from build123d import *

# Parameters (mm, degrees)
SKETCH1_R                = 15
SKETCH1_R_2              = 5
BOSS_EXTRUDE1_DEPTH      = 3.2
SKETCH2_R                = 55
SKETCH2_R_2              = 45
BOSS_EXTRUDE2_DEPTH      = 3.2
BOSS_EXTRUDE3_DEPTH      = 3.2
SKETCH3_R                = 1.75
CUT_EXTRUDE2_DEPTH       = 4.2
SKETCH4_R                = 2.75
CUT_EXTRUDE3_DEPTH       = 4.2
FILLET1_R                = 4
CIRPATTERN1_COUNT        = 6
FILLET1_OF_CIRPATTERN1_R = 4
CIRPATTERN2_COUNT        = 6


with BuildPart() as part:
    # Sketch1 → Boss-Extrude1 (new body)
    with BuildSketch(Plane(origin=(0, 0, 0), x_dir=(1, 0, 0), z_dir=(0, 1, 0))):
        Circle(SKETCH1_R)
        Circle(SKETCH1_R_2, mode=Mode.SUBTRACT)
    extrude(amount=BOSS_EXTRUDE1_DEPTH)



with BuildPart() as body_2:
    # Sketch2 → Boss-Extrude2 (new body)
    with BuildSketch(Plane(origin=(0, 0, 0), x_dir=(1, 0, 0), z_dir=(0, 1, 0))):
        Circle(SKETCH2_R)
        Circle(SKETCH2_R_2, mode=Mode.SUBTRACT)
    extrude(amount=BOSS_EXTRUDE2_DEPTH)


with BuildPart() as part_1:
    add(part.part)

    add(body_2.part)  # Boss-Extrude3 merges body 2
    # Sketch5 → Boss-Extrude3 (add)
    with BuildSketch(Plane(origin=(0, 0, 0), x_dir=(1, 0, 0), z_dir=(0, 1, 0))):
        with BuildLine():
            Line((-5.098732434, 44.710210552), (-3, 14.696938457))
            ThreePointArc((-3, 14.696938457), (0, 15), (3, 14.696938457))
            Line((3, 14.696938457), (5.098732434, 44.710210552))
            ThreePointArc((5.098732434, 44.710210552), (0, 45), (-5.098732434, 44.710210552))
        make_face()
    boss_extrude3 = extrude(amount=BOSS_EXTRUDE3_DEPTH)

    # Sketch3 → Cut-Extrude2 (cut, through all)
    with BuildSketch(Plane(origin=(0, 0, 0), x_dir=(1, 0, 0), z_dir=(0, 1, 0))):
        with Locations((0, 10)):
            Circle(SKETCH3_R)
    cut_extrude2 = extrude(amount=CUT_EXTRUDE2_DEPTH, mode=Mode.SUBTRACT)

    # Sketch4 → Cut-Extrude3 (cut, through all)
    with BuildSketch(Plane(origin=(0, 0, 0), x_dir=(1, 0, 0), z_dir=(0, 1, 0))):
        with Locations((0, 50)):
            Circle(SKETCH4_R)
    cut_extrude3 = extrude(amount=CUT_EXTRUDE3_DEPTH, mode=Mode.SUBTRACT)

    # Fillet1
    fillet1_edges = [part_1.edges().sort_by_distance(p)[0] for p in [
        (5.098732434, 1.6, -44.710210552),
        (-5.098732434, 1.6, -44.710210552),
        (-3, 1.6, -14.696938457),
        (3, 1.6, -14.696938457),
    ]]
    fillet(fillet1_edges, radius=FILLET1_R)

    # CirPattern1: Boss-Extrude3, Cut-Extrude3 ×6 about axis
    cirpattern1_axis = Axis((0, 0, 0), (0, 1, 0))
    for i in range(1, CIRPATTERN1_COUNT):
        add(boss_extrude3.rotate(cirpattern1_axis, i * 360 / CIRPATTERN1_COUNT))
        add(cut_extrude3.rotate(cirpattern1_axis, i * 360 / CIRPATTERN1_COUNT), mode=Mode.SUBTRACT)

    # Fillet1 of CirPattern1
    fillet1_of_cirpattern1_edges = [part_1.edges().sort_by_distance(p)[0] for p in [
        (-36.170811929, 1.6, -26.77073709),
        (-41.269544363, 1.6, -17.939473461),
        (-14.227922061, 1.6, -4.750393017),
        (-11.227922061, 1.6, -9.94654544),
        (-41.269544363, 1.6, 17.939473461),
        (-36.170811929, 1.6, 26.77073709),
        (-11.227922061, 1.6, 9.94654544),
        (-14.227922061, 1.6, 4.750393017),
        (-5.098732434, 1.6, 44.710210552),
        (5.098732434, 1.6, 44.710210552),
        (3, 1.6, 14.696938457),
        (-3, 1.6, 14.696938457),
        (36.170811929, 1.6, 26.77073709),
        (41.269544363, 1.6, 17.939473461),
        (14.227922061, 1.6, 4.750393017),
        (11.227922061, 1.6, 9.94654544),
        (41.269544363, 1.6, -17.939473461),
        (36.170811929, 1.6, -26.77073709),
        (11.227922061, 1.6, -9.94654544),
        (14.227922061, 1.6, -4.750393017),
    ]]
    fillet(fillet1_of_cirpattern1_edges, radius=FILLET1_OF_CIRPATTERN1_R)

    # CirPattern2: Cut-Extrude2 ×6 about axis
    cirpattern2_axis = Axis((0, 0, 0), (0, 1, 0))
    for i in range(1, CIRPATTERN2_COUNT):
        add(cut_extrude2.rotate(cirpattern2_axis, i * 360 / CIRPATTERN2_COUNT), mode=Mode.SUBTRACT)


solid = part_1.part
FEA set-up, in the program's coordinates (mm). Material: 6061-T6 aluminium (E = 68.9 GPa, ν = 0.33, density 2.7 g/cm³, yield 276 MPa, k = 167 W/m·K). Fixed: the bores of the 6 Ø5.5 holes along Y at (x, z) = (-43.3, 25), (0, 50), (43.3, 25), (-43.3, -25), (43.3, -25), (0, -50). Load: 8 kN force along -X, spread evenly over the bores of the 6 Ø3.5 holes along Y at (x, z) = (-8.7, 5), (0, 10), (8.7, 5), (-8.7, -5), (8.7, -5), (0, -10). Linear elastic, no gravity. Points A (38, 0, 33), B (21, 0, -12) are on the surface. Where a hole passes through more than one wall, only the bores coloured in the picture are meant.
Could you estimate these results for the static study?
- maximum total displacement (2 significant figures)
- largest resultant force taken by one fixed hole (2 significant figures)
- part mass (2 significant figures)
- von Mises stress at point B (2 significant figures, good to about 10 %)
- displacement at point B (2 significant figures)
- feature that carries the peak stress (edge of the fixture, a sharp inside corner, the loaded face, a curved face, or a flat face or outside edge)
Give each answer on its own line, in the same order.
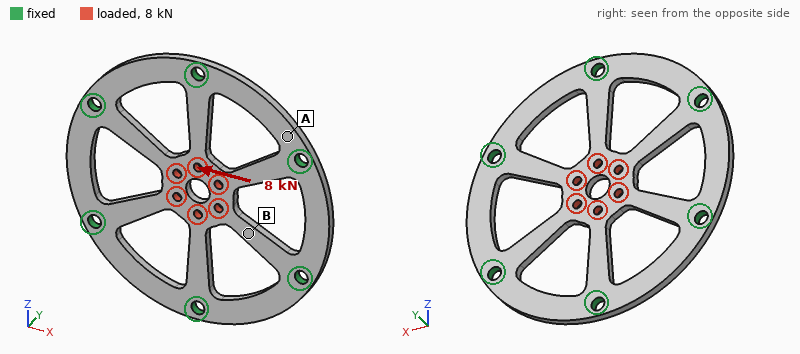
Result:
56 µm
2.1 kN
44 g
93 MPa
31 µm
a sharp inside corner
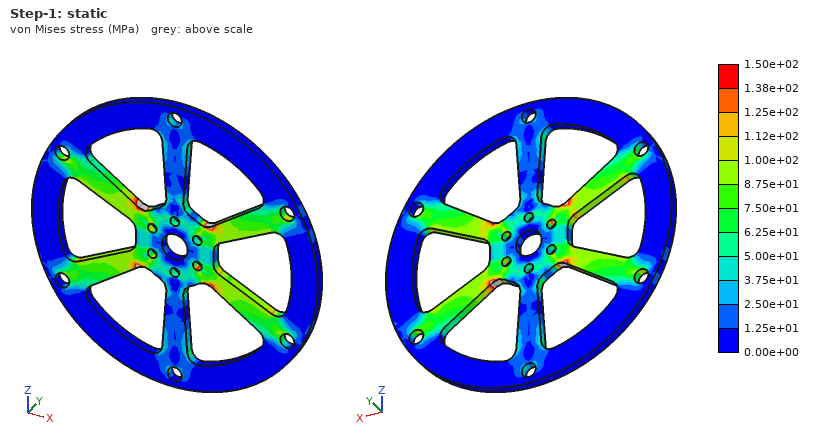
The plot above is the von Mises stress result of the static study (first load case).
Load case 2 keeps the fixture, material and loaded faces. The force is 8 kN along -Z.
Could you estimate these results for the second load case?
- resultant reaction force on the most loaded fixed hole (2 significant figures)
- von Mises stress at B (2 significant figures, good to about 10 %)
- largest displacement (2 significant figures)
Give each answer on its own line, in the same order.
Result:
2.4 kN
55 MPa
55 µm
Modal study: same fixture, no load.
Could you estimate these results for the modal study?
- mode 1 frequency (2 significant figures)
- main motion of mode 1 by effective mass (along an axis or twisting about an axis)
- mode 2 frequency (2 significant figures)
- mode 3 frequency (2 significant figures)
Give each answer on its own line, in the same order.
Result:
2400 Hz
along Y
5500 Hz
5500 Hz
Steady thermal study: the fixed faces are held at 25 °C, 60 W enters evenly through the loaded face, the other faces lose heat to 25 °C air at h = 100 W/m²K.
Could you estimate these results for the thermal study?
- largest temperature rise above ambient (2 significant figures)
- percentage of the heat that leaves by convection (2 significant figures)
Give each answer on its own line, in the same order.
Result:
67 K
33 %
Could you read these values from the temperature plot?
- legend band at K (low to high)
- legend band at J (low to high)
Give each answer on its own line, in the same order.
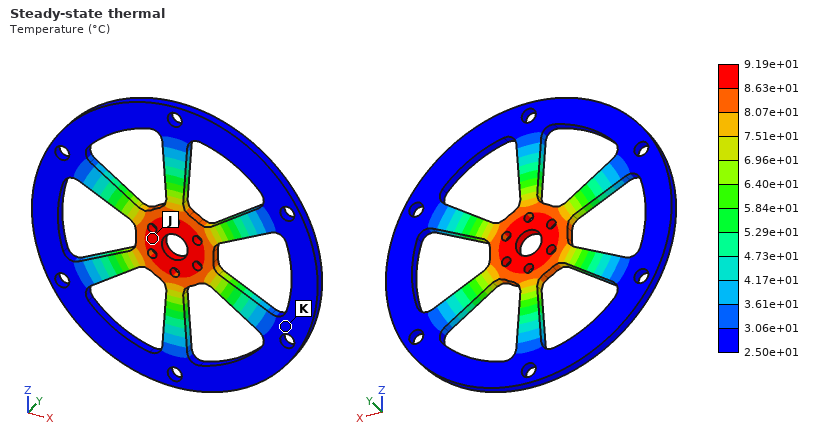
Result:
2.50e+01 to 3.06e+01 °C
8.63e+01 to 9.19e+01 °C
